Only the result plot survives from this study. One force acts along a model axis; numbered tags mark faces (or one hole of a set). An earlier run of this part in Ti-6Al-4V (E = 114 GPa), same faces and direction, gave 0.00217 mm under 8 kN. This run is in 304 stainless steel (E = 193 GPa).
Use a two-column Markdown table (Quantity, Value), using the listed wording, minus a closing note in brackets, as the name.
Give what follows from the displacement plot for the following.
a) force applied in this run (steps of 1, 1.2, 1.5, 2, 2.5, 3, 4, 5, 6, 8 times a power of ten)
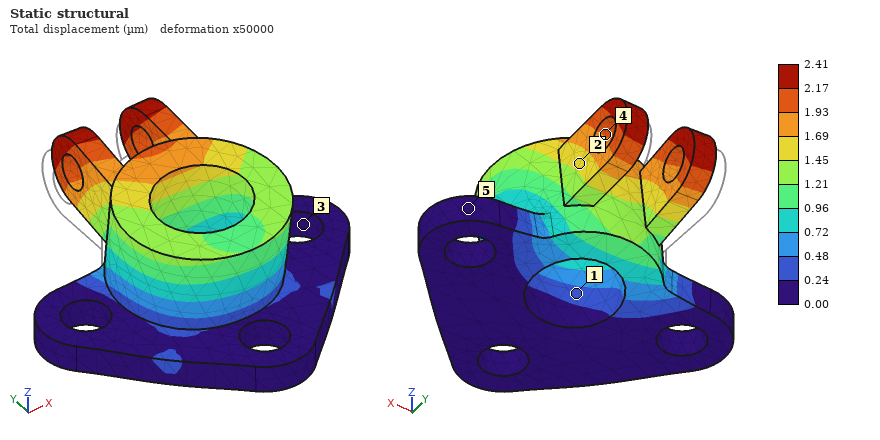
| Quantity | Value |
|---|---|
| force applied in this run | 15 kN |
